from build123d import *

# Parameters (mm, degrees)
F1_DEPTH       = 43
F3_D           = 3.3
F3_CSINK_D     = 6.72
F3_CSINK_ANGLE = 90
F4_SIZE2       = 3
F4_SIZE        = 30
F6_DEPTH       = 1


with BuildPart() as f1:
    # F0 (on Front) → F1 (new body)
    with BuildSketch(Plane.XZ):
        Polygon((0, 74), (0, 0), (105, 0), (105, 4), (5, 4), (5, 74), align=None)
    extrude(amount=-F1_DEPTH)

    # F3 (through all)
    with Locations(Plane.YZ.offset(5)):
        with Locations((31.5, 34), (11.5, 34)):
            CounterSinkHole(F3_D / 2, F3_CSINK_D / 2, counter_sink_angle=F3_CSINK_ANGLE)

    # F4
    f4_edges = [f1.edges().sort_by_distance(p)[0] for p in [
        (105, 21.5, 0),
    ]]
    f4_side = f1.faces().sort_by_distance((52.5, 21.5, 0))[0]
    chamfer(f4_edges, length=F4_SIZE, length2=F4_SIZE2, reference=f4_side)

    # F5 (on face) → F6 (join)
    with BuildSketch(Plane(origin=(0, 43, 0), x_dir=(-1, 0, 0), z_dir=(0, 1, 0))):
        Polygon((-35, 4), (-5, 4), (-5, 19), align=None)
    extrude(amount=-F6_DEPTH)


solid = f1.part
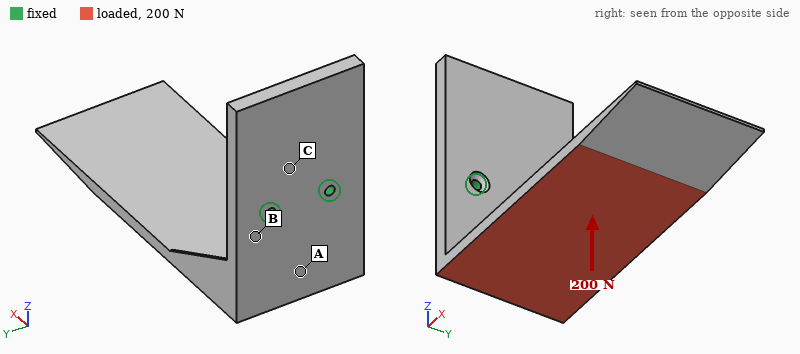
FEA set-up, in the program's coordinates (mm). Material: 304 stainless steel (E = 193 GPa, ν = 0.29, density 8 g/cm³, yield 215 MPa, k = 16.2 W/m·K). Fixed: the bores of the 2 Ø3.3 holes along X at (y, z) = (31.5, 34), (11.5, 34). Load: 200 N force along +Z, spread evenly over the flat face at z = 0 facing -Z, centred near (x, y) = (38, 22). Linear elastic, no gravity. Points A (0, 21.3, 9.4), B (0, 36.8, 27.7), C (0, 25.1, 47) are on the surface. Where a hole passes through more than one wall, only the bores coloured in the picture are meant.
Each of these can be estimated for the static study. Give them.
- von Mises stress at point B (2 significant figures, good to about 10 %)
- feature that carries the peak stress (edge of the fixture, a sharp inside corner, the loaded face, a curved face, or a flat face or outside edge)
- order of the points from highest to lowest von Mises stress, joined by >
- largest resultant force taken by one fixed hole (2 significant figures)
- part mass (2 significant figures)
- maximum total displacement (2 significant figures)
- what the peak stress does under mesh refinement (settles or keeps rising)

41 MPa
edge of the fixture
B > A > C
110 N
250 g
0.49 mm
keeps rising
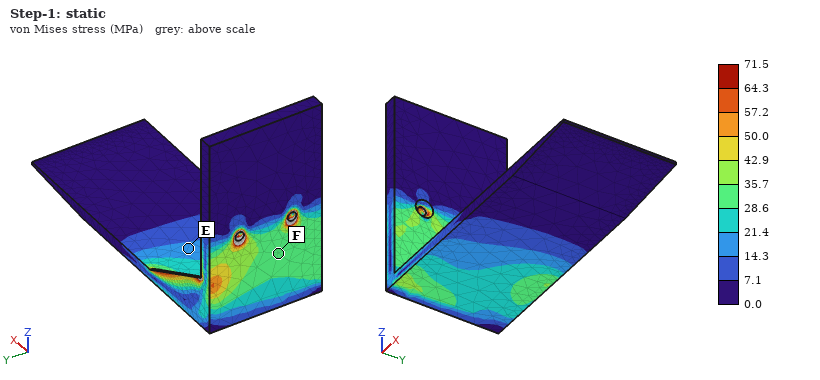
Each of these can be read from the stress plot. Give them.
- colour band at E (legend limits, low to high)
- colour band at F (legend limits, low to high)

14.3 to 21.4 MPa
28.6 to 35.7 MPa
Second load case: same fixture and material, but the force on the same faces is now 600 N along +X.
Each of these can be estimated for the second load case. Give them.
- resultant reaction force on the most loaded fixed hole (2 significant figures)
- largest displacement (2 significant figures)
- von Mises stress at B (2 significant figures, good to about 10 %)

310 N
0.57 mm
87 MPa
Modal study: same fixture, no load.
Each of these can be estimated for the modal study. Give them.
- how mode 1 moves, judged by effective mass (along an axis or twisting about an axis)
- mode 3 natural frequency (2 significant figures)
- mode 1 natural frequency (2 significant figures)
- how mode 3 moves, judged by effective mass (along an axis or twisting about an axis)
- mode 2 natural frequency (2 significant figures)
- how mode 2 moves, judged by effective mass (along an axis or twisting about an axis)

along Z
1200 Hz
310 Hz
along X
620 Hz
along Y
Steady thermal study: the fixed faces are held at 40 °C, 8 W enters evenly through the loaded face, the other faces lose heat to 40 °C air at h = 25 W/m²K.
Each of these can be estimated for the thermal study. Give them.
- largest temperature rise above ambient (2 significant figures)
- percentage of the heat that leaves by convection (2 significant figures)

40 K
77 %
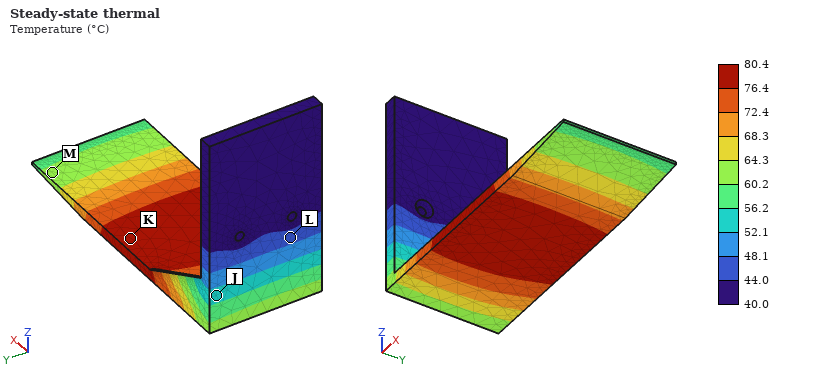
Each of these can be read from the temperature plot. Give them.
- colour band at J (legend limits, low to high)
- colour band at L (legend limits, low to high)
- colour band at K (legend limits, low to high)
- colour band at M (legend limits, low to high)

52.1 to 56.2 °C
44.0 to 48.1 °C
76.4 to 80.4 °C
60.2 to 64.3 °C
